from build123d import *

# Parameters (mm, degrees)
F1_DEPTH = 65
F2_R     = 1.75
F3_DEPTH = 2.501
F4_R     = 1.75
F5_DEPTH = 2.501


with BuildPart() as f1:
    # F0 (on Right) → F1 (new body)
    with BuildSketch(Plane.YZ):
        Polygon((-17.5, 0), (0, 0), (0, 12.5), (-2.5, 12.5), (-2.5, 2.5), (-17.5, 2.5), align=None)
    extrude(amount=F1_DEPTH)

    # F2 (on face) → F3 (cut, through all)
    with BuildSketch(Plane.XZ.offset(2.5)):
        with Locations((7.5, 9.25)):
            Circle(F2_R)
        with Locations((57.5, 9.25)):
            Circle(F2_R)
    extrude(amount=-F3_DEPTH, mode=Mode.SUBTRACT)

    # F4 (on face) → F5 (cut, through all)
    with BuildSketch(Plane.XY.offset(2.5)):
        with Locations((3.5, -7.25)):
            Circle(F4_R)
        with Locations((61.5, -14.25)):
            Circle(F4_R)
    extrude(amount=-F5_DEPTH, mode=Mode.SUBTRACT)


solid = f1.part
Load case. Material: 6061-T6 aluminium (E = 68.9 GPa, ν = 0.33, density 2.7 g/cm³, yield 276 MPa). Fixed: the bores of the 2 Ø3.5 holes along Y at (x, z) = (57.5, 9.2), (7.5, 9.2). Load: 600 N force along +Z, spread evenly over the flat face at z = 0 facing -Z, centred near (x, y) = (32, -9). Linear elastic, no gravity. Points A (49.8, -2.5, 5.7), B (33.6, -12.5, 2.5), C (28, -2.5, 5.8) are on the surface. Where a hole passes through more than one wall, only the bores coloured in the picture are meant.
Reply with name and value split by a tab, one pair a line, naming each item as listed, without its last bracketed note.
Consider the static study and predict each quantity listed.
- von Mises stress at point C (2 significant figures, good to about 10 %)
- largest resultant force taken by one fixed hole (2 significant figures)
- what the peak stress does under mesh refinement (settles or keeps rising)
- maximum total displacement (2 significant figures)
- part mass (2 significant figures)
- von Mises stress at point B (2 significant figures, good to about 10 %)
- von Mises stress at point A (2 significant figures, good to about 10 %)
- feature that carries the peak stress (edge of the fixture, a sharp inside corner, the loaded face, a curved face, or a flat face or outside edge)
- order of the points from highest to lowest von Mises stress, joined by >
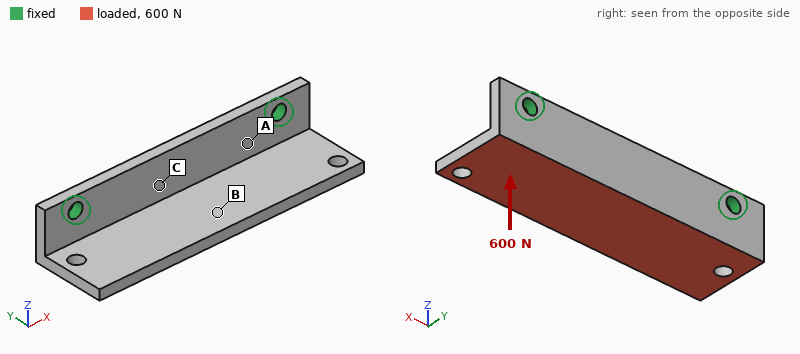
von Mises stress at point C	28 MPa
largest resultant force taken by one fixed hole	330 N
what the peak stress does under mesh refinement	keeps rising
maximum total displacement	0.24 mm
part mass	12 g
von Mises stress at point B	15 MPa
von Mises stress at point A	78 MPa
feature that carries the peak stress	edge of the fixture
order of the points from highest to lowest von Mises stress, joined by >	A > C > B
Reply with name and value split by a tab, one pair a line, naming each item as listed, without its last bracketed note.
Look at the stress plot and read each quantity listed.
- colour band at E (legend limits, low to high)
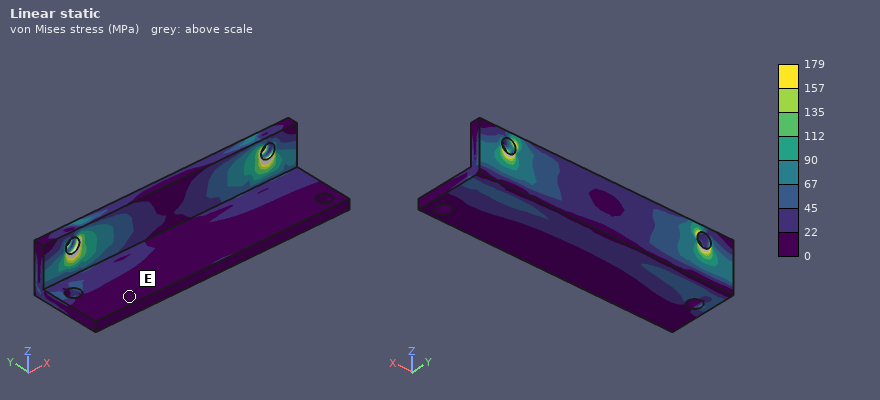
colour band at E	0 to 22 MPa
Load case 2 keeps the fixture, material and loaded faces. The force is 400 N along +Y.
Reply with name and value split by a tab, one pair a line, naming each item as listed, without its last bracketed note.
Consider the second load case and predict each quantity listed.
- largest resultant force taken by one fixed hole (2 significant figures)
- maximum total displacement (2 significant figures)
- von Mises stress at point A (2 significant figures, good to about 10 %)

largest resultant force taken by one fixed hole	200 N
maximum total displacement	94 µm
von Mises stress at point A	26 MPa
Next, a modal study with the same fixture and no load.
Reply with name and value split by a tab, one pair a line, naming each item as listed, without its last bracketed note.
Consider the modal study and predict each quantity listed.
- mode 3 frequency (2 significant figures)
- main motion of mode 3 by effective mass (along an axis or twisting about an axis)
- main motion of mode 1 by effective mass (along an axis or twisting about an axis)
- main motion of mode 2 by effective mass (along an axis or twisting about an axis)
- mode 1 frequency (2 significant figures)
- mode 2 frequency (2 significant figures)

mode 3 frequency	8100 Hz
main motion of mode 3 by effective mass	along Y
main motion of mode 1 by effective mass	along Z
main motion of mode 2 by effective mass	twisting about Y
mode 1 frequency	3500 Hz
mode 2 frequency	5800 Hz
